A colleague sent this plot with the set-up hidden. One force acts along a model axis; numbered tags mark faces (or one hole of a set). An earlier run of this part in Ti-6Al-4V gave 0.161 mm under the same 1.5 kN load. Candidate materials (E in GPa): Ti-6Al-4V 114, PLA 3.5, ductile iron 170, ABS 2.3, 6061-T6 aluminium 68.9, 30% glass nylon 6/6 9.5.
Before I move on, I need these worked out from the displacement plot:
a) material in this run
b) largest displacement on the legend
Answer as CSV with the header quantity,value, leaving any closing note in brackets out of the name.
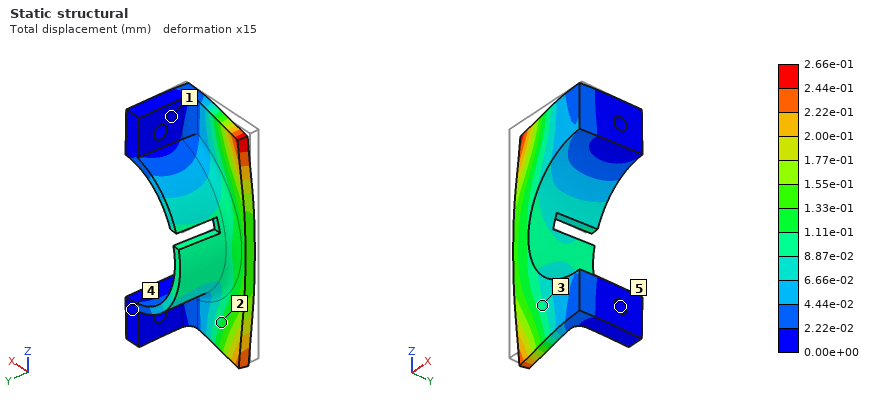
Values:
quantity,value
material in this run,6061-T6 aluminium
largest displacement on the legend,2.66e-01 mm
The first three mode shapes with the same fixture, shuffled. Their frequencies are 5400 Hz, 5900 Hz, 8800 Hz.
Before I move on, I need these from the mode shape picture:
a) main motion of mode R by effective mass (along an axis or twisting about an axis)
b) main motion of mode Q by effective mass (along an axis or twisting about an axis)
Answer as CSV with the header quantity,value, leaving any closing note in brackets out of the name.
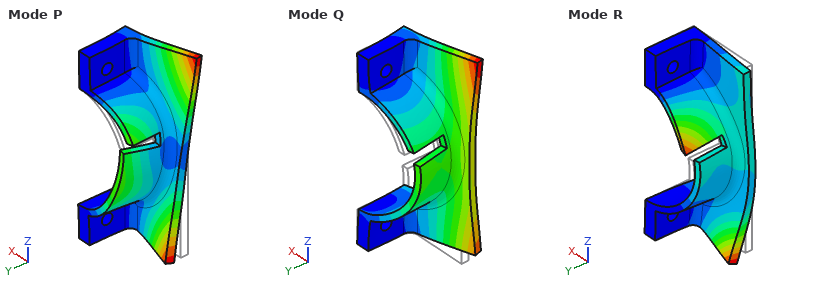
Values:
quantity,value
main motion of mode R by effective mass,along Z
main motion of mode Q by effective mass,along Y
